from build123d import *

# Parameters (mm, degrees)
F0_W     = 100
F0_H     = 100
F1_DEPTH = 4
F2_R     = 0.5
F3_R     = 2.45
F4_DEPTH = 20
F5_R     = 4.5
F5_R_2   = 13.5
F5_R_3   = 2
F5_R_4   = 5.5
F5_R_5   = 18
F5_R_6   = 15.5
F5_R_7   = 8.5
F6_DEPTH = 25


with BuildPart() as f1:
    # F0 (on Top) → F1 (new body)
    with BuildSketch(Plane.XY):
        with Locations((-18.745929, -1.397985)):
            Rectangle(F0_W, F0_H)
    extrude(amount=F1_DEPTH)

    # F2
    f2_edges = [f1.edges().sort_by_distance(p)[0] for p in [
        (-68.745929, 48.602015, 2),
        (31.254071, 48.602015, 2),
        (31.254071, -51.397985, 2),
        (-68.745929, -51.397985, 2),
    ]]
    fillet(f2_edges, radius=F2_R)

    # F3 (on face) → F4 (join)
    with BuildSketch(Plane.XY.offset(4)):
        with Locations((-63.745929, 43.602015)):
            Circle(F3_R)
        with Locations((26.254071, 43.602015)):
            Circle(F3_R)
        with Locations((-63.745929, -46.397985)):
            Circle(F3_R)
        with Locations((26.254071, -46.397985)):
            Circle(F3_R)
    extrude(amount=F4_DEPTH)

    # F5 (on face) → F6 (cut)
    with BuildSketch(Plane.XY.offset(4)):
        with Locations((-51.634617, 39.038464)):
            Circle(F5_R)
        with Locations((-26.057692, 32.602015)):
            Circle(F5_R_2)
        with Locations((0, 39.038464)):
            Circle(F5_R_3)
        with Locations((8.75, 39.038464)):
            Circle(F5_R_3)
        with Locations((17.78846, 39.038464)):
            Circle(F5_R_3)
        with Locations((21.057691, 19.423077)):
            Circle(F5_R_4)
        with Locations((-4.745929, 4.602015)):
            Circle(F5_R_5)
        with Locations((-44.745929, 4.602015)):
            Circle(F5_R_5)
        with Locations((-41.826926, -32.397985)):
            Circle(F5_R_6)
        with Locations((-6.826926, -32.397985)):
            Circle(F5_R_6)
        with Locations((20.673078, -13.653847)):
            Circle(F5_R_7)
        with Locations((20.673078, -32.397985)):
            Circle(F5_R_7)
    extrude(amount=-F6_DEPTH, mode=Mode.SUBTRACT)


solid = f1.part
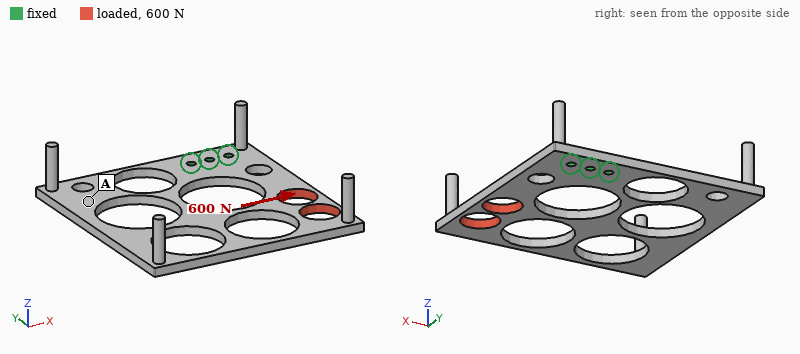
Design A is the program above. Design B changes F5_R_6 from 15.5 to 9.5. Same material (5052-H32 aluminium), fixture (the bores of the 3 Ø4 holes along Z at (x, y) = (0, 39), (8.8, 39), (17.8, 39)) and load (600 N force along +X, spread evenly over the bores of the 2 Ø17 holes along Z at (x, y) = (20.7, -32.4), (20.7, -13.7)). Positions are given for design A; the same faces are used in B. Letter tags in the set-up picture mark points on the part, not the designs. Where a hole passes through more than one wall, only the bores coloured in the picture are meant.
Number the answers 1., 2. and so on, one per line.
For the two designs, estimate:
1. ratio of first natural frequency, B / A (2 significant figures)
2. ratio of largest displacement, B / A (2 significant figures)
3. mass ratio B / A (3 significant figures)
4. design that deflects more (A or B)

1. 0.89
2. 0.84
3. 1.17
4. A
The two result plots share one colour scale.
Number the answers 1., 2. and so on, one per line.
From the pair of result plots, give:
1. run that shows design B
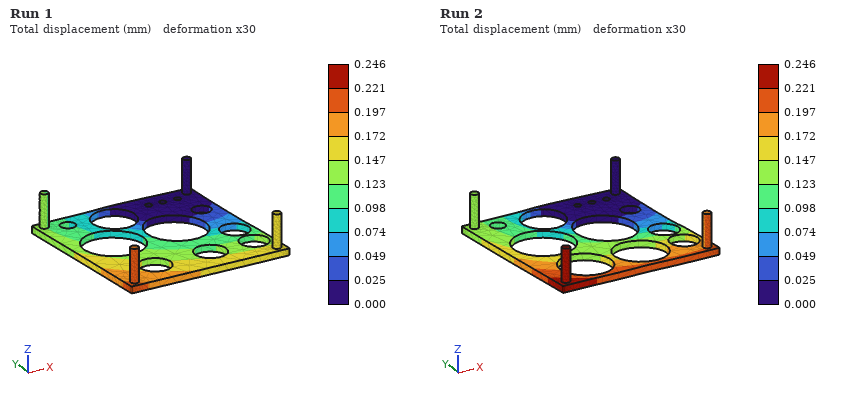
1. Run 1
